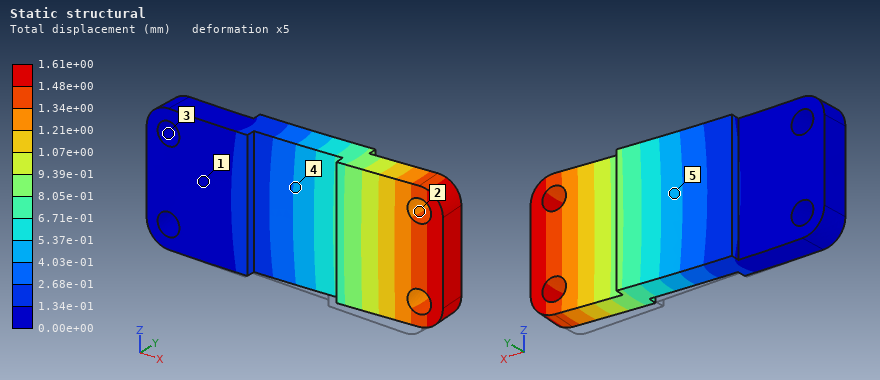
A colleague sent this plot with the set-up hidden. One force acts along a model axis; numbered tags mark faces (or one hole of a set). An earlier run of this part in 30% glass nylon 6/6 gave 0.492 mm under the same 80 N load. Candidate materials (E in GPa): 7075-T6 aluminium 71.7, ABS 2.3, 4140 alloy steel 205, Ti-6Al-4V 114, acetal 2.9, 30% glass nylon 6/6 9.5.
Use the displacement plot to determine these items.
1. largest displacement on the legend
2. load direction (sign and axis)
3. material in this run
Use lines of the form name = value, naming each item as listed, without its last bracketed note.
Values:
largest displacement on the legend = 1.61e+00 mm
load direction = +Y
material in this run = acetal
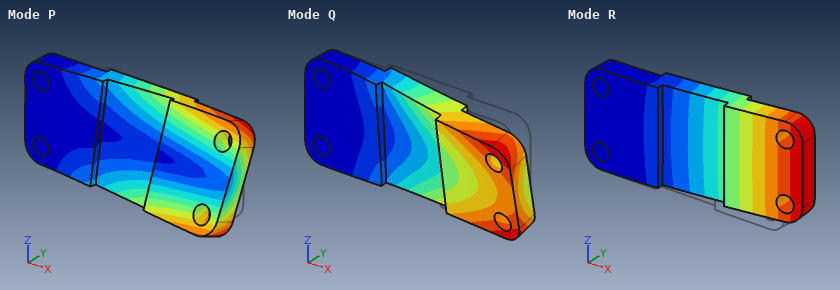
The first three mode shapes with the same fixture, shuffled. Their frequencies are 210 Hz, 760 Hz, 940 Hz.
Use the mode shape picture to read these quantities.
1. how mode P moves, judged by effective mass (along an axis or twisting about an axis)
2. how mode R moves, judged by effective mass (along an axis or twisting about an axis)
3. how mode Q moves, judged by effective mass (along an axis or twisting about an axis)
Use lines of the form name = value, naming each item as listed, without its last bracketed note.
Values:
how mode P moves, judged by effective mass = along Z
how mode R moves, judged by effective mass = along Y
how mode Q moves, judged by effective mass = along Z
